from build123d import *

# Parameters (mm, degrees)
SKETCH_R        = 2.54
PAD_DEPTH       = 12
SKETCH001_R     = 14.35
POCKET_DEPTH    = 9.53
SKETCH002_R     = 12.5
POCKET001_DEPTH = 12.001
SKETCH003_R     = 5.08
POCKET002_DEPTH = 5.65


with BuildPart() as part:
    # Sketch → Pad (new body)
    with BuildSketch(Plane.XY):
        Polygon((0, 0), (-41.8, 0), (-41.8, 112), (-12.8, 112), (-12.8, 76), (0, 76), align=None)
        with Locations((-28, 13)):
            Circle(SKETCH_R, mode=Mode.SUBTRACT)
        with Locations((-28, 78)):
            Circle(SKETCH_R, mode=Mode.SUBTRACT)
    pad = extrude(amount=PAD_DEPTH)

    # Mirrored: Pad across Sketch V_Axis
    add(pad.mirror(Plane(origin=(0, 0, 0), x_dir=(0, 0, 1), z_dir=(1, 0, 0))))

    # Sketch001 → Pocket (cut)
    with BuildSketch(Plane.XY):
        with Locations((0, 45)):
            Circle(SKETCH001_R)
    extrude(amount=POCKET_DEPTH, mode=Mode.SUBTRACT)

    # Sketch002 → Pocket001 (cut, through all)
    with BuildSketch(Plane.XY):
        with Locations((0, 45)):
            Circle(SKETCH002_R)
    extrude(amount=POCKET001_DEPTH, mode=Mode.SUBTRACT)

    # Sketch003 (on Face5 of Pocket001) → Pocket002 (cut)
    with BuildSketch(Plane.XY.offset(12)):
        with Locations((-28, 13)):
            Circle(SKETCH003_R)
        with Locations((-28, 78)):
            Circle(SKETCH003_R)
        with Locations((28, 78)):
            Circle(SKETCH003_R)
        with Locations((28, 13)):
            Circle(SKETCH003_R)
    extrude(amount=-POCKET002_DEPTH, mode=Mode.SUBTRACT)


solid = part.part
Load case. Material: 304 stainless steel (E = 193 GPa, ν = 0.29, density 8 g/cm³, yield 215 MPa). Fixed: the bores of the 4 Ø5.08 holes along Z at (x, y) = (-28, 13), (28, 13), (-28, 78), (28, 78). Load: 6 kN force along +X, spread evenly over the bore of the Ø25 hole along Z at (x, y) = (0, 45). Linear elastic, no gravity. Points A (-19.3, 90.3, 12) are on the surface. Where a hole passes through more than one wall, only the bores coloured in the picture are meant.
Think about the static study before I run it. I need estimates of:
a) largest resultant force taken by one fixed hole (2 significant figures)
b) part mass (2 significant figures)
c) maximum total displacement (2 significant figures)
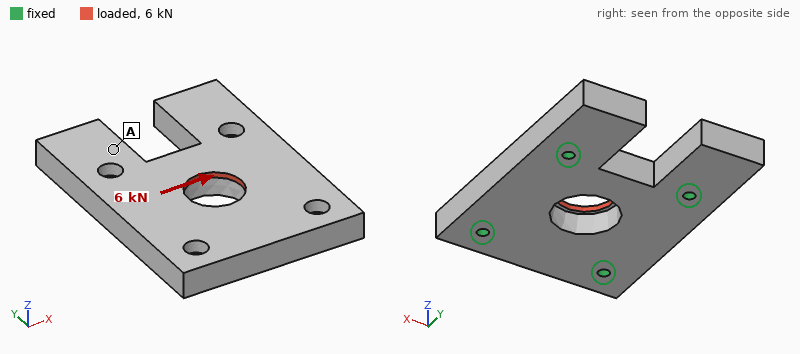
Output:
1.8 kN
730 g
3.9 µm
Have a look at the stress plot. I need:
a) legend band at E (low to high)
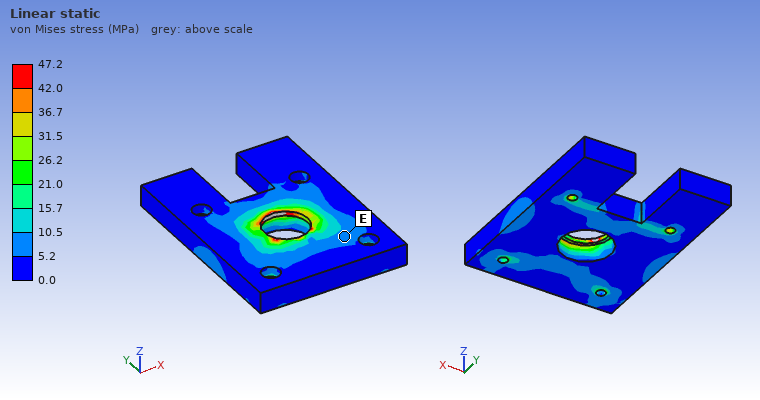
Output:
5.2 to 10.5 MPa
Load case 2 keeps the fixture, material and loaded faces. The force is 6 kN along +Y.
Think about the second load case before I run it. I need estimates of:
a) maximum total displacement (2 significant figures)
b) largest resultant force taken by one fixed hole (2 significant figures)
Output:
3.7 µm
1.7 kN
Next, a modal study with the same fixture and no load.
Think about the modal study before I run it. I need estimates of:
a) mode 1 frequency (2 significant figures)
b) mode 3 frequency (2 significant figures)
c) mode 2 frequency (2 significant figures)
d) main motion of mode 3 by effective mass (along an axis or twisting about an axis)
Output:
5100 Hz
7900 Hz
5300 Hz
along Z
